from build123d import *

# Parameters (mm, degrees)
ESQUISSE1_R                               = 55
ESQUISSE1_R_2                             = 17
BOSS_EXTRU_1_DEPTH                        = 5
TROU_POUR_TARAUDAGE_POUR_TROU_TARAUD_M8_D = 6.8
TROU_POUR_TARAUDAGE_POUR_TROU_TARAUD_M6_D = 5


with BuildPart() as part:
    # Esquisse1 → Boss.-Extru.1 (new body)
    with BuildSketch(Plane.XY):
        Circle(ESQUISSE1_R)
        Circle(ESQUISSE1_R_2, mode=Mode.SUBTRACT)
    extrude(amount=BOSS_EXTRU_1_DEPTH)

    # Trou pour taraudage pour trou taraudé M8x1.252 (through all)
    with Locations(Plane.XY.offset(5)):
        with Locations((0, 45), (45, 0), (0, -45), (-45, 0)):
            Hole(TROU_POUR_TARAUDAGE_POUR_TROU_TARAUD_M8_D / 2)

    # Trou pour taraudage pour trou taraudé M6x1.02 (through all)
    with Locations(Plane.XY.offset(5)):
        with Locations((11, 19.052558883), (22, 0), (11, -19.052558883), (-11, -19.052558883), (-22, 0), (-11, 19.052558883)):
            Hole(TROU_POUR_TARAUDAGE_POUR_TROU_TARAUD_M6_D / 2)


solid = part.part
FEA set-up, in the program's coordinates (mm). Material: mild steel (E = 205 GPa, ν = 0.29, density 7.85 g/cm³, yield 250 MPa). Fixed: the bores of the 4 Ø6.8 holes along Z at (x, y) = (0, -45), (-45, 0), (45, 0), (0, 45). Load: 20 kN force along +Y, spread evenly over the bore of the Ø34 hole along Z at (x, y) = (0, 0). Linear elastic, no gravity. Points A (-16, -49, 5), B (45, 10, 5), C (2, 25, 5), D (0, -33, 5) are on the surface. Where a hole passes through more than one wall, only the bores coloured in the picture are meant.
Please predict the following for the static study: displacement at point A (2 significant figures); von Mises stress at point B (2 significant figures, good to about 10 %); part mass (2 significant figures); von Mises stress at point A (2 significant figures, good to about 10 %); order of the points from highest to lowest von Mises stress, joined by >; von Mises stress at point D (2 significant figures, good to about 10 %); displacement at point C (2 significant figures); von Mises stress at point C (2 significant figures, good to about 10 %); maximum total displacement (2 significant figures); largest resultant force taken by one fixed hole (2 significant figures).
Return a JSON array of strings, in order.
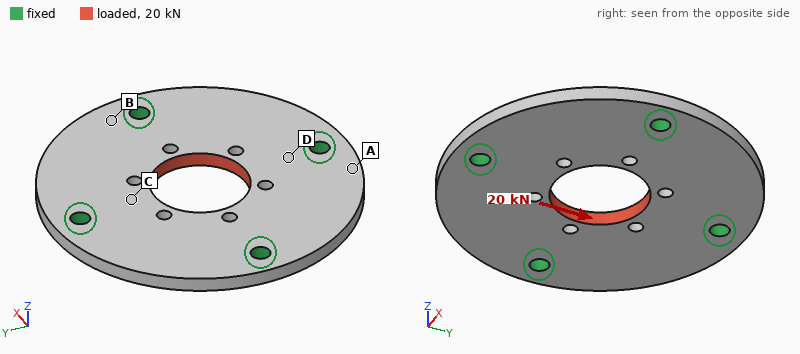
["3.3 µm", "25 MPa", "330 g", "12 MPa", "D > C > B > A", "67 MPa", "5.3 µm", "54 MPa", "9.9 µm", "6.0 kN"]
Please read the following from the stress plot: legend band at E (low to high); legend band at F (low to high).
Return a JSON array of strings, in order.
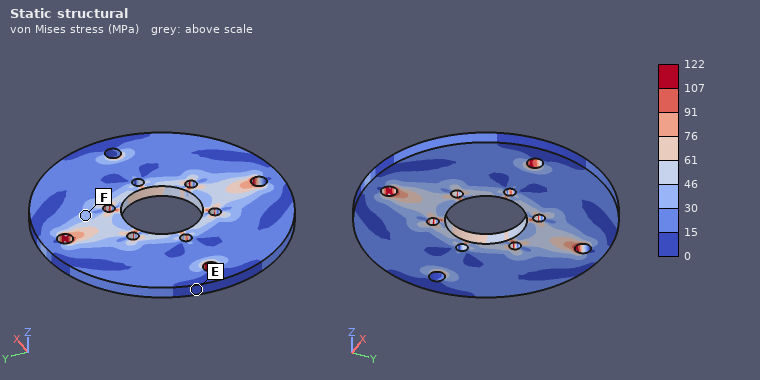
["0 to 15 MPa", "30 to 46 MPa"]
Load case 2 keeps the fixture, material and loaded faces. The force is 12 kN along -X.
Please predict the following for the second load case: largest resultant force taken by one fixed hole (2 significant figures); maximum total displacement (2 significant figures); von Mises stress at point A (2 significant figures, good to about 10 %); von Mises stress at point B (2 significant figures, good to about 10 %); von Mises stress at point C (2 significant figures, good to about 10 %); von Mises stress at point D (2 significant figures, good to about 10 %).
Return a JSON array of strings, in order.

["3.6 kN", "6.0 µm", "9.0 MPa", "16 MPa", "11 MPa", "7.4 MPa"]
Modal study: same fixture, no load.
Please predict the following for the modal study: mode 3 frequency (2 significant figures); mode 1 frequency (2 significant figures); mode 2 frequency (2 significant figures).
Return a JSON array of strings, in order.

["5300 Hz", "5000 Hz", "5300 Hz"]
